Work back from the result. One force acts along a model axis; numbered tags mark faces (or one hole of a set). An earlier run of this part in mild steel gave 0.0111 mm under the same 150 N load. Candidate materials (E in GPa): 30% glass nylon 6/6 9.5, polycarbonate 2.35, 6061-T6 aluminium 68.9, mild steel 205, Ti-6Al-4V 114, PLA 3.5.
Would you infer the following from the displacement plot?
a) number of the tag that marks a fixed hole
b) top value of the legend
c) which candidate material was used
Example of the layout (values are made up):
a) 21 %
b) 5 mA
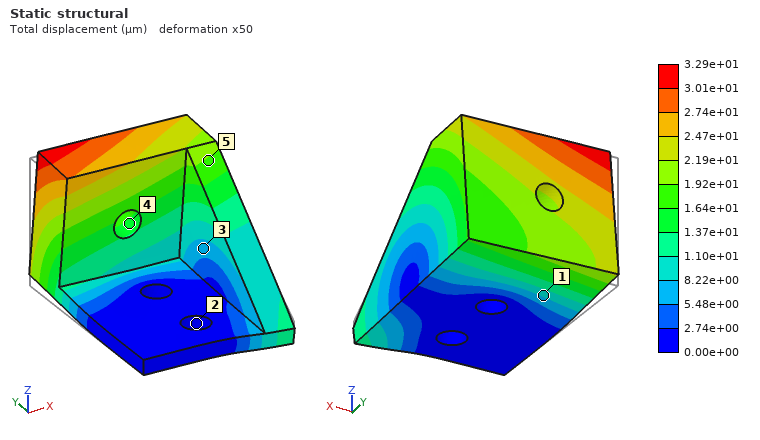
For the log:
a) 2
b) 3.29e+01 µm
c) 6061-T6 aluminium
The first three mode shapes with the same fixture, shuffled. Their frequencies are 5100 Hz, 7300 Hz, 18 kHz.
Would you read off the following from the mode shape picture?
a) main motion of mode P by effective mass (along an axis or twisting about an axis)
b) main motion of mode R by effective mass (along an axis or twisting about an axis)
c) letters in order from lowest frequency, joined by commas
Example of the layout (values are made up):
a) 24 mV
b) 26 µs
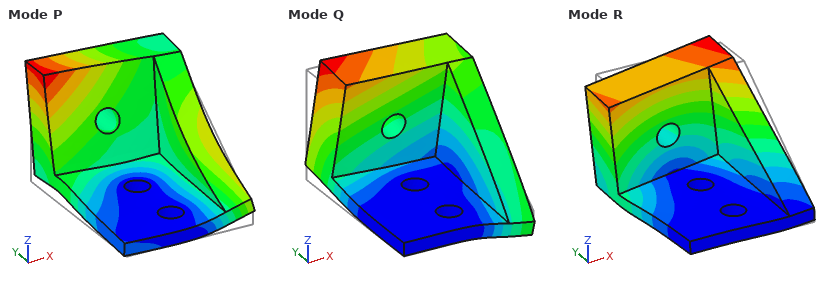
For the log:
a) along Z
b) along X
c) R, Q, P
